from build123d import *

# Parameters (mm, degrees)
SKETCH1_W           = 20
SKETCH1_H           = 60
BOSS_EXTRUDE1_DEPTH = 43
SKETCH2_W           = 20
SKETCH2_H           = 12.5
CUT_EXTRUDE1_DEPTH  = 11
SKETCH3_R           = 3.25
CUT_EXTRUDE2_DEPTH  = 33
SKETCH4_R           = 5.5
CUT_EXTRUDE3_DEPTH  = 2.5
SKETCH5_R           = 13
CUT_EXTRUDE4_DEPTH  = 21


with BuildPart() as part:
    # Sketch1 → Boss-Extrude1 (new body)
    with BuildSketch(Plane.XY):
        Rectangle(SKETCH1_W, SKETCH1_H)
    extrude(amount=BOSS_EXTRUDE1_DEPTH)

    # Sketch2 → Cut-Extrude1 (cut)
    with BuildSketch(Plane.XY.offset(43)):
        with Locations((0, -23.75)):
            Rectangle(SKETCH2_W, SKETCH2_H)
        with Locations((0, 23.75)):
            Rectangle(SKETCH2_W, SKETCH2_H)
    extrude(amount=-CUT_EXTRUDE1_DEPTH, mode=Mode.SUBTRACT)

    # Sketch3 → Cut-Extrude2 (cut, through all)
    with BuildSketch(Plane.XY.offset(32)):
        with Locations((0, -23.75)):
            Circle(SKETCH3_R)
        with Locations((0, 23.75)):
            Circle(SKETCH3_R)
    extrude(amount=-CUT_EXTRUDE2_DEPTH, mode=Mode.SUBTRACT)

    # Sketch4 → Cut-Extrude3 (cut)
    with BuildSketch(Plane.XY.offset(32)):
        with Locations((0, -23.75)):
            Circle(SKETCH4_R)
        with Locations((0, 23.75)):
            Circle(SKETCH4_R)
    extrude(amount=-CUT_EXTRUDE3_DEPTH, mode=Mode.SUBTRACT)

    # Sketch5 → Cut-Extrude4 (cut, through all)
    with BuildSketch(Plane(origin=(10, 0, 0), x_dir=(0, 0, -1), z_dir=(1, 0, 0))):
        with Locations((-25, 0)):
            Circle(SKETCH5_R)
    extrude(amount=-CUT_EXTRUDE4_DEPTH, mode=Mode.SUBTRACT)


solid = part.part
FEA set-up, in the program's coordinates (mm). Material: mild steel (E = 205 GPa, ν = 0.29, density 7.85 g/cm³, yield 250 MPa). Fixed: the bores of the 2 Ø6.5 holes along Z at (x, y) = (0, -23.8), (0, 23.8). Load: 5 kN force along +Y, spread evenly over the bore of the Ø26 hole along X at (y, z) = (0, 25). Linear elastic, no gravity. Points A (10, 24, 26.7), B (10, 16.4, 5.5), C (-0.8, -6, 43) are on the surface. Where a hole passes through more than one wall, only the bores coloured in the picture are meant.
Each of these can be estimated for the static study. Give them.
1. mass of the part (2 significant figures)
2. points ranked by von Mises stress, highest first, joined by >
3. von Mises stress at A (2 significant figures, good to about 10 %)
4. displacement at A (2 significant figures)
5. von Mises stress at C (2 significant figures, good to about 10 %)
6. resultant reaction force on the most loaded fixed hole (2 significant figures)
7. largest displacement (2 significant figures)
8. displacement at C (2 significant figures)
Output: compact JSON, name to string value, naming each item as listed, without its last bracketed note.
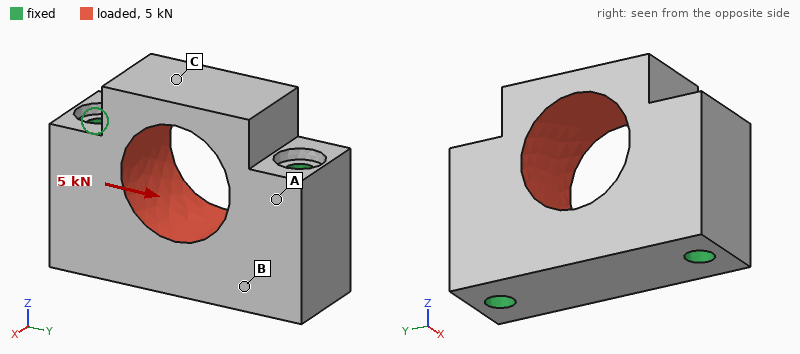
{"mass of the part": "260 g", "points ranked by von Mises stress, highest first, joined by >": "C > A > B", "von Mises stress at A": "5.0 MPa", "displacement at A": "0.39 µm", "von Mises stress at C": "10 MPa", "resultant reaction force on the most loaded fixed hole": "2.5 kN", "largest displacement": "2.4 µm", "displacement at C": "2.0 µm"}
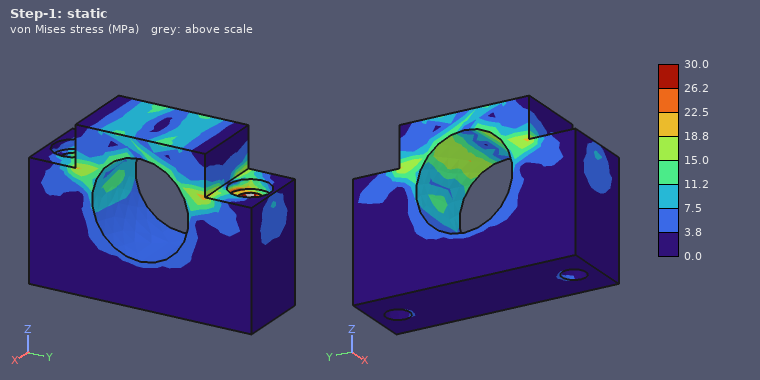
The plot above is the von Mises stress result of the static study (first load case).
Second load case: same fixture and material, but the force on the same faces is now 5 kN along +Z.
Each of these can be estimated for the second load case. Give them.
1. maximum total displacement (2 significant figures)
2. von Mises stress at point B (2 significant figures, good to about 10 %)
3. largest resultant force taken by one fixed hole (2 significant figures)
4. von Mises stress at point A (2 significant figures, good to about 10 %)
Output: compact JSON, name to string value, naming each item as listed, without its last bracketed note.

{"maximum total displacement": "2.0 µm", "von Mises stress at point B": "3.5 MPa", "largest resultant force taken by one fixed hole": "2.5 kN", "von Mises stress at point A": "2.9 MPa"}
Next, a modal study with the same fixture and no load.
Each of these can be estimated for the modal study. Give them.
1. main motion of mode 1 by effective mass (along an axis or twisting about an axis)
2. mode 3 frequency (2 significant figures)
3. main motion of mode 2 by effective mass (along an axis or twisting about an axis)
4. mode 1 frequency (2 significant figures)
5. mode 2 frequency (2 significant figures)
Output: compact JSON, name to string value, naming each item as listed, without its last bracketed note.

{"main motion of mode 1 by effective mass": "along X", "mode 3 frequency": "24 kHz", "main motion of mode 2 by effective mass": "along Y", "mode 1 frequency": "15 kHz", "mode 2 frequency": "22 kHz"}
